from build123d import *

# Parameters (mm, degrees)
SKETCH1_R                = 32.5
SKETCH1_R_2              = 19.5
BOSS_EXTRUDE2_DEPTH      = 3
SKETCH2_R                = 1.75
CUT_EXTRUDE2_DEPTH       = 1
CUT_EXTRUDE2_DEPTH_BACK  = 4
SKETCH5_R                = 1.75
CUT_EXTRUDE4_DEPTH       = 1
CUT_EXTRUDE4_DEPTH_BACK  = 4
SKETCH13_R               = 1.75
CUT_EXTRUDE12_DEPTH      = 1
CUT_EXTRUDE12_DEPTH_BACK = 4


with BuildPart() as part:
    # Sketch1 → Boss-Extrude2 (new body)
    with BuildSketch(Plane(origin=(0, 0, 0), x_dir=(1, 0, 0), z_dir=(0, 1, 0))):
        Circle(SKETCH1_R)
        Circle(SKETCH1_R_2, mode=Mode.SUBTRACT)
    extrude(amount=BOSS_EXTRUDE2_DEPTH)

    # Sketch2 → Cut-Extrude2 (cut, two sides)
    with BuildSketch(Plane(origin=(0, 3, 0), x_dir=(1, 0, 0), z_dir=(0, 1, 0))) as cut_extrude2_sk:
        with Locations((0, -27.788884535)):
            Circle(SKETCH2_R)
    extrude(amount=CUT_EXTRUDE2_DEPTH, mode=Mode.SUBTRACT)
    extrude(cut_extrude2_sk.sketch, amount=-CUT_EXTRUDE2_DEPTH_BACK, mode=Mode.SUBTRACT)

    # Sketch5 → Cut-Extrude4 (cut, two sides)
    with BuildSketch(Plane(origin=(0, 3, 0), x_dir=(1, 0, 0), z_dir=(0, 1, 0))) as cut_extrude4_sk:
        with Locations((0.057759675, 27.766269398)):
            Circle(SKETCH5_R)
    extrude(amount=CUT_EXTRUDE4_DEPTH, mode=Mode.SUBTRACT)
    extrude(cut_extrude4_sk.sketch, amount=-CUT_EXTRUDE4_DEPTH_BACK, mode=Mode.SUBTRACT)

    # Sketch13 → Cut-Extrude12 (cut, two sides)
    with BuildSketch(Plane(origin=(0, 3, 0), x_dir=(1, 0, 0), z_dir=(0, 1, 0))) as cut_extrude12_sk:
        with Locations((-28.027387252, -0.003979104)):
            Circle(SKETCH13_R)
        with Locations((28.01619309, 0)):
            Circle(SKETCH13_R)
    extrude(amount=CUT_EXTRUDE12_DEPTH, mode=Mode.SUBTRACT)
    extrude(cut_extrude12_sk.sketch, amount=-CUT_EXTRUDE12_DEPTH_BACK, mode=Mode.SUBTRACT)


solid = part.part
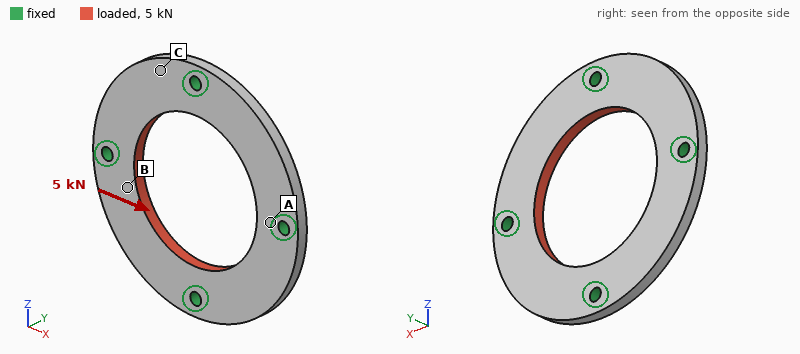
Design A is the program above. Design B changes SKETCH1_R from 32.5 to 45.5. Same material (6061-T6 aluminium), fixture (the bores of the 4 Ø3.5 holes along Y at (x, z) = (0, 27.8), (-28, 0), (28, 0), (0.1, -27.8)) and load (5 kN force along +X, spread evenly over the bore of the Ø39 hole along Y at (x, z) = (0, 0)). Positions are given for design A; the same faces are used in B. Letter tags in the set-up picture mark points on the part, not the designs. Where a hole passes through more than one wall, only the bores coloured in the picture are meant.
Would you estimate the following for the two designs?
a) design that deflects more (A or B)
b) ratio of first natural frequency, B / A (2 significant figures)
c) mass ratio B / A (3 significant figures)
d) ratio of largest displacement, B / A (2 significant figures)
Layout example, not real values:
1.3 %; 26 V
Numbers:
A; 0.43; 2.53; 0.62
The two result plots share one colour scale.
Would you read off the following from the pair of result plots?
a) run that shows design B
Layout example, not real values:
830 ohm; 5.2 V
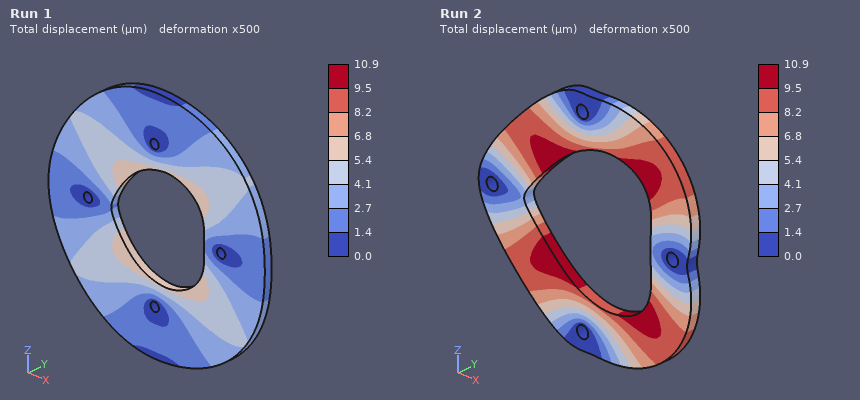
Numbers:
Run 1
